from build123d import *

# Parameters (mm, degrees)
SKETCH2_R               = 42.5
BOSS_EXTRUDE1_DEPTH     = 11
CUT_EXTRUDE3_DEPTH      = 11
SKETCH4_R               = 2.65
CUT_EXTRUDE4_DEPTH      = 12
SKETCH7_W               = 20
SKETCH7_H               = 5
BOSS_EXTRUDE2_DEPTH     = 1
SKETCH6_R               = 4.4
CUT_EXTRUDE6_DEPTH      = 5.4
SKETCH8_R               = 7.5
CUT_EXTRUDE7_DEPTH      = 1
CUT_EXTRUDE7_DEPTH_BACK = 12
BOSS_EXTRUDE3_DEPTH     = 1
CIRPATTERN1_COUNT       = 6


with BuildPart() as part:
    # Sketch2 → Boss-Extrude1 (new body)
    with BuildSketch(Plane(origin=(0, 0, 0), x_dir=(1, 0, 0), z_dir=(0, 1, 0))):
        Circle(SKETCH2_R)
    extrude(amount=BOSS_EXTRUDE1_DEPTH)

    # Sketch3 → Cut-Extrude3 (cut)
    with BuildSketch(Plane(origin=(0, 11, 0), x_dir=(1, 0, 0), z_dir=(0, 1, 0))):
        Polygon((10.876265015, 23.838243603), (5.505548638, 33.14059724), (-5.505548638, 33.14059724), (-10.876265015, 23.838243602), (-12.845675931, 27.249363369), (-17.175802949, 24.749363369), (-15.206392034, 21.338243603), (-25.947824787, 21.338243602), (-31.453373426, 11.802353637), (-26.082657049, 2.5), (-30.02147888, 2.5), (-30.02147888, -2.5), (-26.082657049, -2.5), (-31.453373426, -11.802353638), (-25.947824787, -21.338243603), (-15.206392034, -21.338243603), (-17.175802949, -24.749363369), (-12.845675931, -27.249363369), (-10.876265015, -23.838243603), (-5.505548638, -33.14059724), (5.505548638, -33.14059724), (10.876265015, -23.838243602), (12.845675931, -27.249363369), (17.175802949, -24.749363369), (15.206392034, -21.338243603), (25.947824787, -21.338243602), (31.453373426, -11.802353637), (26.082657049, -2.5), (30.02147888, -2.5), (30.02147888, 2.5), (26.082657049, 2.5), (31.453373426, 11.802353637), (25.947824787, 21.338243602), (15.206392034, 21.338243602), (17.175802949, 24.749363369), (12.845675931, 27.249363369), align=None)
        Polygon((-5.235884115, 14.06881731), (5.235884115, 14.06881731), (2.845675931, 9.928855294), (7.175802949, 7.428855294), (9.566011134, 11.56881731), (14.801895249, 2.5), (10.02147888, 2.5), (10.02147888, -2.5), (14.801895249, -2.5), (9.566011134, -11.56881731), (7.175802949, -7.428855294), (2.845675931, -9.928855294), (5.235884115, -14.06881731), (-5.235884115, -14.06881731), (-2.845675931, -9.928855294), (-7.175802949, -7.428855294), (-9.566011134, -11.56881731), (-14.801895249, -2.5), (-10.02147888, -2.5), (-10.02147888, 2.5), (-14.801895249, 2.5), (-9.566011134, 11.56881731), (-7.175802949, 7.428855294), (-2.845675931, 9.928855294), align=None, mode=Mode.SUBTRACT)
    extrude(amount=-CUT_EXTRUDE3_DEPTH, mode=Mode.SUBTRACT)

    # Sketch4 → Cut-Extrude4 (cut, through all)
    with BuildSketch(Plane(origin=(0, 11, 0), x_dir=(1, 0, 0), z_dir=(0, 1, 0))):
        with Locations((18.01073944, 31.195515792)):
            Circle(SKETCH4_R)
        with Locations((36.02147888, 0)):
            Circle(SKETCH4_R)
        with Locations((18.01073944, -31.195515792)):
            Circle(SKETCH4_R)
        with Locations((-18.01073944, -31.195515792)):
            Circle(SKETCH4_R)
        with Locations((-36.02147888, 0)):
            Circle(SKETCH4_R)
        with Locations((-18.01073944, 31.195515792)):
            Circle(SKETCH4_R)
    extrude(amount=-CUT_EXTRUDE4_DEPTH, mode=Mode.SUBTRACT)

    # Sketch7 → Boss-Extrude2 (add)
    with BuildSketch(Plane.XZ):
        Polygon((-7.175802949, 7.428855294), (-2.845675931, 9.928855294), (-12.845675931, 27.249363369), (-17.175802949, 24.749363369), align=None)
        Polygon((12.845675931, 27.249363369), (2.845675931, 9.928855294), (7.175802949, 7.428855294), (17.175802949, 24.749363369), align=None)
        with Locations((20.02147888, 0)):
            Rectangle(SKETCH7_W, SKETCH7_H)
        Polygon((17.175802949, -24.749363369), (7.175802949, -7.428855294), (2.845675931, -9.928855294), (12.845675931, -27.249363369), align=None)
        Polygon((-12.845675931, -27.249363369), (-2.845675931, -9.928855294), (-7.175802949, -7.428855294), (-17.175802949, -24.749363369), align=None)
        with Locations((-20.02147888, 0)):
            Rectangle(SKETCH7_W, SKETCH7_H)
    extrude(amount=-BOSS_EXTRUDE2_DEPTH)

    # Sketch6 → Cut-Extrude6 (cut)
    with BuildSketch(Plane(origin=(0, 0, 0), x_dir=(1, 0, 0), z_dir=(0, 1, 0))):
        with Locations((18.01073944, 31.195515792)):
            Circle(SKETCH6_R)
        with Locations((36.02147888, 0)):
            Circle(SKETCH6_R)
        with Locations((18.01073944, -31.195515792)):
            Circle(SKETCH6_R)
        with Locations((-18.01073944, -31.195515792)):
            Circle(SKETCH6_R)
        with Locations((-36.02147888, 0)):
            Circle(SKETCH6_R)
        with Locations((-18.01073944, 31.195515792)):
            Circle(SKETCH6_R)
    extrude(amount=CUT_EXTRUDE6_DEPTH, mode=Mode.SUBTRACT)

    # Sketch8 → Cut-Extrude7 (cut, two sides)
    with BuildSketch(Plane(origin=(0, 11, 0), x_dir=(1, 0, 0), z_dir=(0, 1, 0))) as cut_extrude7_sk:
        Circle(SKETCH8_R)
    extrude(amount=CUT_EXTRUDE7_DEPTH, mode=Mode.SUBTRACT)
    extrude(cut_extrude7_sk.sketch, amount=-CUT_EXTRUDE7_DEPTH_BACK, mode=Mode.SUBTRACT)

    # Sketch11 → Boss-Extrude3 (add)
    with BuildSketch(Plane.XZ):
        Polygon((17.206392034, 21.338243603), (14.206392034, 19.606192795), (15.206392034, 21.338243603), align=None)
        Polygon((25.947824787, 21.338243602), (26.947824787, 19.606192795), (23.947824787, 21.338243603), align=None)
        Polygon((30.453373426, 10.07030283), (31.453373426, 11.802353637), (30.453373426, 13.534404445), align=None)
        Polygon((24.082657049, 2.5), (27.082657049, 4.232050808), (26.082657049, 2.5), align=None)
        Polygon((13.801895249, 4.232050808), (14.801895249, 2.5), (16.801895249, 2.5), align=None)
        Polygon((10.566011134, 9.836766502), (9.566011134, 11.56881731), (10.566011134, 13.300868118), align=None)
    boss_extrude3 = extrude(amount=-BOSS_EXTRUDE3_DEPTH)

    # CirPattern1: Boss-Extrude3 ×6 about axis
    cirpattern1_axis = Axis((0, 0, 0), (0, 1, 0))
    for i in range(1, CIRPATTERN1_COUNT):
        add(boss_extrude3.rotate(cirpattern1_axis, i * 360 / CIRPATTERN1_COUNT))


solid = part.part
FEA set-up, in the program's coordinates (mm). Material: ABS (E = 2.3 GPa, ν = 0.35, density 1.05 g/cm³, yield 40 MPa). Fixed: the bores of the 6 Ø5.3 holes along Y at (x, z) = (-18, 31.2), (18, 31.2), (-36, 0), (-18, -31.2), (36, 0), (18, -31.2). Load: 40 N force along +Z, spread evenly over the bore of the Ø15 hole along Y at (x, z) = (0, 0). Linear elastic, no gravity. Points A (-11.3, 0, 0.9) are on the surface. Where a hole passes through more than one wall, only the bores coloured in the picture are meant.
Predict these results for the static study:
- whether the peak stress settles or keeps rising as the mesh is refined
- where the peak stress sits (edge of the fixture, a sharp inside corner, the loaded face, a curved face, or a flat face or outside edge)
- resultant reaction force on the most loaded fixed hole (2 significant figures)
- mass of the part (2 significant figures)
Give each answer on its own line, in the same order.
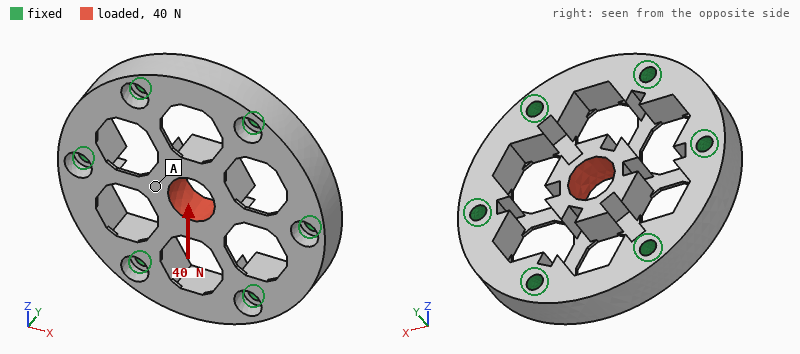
keeps rising
a sharp inside corner
8.1 N
33 g
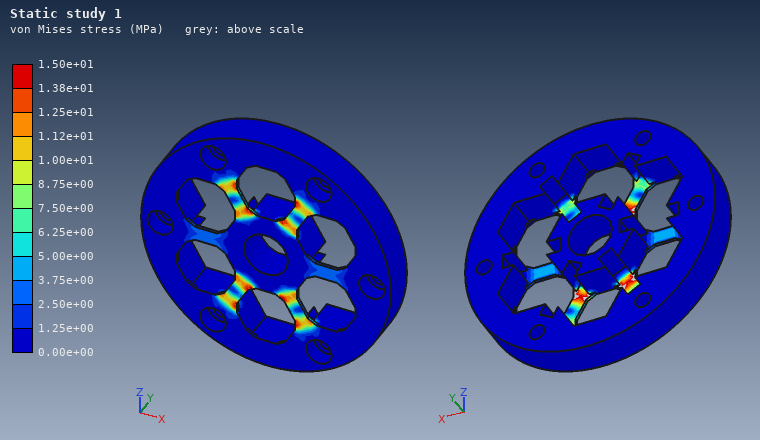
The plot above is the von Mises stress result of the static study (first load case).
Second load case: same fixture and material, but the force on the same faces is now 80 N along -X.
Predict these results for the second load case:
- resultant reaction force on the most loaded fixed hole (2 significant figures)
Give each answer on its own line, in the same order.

18 N
